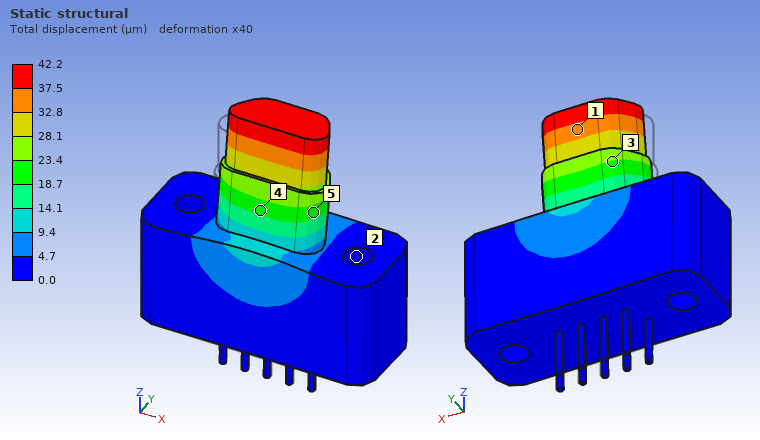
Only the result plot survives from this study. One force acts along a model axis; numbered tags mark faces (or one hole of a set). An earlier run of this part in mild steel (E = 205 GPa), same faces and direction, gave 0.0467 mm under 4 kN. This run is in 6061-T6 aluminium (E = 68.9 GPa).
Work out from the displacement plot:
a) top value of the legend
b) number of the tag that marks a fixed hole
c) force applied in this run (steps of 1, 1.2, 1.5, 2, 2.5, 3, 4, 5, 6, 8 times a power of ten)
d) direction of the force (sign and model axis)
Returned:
42.2 µm
2
1.2 kN
+Y
